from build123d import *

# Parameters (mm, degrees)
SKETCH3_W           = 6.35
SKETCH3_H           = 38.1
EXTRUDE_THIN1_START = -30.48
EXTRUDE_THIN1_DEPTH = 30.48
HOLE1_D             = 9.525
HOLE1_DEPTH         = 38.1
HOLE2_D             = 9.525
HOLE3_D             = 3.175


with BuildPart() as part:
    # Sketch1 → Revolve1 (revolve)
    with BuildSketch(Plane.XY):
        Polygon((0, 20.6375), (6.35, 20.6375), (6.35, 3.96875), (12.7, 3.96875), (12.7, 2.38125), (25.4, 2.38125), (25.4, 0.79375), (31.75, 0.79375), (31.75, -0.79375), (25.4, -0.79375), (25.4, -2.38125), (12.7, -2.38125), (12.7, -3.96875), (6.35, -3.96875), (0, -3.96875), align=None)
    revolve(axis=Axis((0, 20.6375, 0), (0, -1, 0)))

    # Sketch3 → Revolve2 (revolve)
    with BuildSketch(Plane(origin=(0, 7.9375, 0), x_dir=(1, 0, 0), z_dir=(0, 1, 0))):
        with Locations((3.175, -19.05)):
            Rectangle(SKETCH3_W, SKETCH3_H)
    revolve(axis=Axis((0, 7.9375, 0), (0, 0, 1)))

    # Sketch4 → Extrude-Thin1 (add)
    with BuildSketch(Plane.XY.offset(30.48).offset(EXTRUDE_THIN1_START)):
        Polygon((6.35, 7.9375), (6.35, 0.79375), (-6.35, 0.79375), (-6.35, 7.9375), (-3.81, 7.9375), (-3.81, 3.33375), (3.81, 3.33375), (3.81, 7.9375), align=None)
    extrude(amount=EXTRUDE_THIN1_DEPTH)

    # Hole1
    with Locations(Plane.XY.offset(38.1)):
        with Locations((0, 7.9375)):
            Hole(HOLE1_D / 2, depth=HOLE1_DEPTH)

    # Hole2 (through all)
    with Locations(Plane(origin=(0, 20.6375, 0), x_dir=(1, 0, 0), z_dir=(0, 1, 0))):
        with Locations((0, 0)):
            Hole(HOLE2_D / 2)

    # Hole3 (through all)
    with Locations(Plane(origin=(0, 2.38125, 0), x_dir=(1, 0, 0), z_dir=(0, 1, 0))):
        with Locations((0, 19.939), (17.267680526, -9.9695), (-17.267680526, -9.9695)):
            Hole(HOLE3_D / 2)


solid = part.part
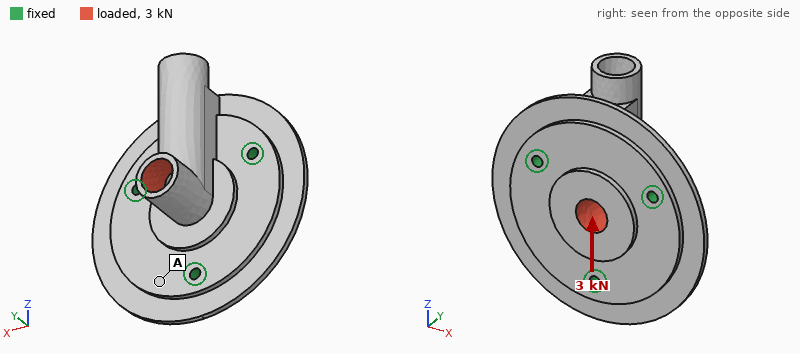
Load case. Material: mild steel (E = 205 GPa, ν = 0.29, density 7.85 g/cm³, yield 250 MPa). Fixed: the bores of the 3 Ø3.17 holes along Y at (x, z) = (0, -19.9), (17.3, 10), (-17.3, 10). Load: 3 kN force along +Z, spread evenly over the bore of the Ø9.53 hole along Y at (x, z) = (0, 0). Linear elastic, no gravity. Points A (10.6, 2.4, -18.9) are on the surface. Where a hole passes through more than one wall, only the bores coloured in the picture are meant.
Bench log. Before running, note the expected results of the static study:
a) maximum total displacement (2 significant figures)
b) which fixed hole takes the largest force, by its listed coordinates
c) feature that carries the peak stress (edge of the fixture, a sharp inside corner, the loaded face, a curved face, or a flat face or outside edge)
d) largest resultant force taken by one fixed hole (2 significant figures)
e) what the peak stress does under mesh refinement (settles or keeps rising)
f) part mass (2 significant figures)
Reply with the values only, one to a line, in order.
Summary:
22 µm
(0, -19.9)
edge of the fixture
1.3 kN
keeps rising
120 g
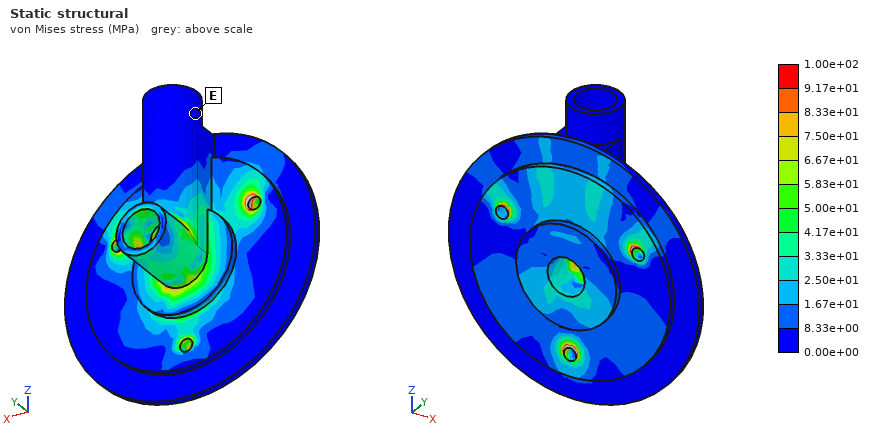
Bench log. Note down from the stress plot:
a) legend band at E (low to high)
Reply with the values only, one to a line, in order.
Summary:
0.00e+00 to 8.33e+00 MPa
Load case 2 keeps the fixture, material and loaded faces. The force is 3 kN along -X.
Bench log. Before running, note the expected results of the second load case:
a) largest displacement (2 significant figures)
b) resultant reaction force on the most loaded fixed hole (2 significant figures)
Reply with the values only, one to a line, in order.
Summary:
24 µm
1.3 kN
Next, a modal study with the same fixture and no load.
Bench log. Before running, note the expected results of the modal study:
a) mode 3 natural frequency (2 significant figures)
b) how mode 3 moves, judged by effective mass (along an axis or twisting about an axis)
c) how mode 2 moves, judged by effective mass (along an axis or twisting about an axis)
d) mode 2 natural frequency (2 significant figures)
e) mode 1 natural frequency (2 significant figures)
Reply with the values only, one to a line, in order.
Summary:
11 kHz
along Y
twisting about Z
10 kHz
7600 Hz
